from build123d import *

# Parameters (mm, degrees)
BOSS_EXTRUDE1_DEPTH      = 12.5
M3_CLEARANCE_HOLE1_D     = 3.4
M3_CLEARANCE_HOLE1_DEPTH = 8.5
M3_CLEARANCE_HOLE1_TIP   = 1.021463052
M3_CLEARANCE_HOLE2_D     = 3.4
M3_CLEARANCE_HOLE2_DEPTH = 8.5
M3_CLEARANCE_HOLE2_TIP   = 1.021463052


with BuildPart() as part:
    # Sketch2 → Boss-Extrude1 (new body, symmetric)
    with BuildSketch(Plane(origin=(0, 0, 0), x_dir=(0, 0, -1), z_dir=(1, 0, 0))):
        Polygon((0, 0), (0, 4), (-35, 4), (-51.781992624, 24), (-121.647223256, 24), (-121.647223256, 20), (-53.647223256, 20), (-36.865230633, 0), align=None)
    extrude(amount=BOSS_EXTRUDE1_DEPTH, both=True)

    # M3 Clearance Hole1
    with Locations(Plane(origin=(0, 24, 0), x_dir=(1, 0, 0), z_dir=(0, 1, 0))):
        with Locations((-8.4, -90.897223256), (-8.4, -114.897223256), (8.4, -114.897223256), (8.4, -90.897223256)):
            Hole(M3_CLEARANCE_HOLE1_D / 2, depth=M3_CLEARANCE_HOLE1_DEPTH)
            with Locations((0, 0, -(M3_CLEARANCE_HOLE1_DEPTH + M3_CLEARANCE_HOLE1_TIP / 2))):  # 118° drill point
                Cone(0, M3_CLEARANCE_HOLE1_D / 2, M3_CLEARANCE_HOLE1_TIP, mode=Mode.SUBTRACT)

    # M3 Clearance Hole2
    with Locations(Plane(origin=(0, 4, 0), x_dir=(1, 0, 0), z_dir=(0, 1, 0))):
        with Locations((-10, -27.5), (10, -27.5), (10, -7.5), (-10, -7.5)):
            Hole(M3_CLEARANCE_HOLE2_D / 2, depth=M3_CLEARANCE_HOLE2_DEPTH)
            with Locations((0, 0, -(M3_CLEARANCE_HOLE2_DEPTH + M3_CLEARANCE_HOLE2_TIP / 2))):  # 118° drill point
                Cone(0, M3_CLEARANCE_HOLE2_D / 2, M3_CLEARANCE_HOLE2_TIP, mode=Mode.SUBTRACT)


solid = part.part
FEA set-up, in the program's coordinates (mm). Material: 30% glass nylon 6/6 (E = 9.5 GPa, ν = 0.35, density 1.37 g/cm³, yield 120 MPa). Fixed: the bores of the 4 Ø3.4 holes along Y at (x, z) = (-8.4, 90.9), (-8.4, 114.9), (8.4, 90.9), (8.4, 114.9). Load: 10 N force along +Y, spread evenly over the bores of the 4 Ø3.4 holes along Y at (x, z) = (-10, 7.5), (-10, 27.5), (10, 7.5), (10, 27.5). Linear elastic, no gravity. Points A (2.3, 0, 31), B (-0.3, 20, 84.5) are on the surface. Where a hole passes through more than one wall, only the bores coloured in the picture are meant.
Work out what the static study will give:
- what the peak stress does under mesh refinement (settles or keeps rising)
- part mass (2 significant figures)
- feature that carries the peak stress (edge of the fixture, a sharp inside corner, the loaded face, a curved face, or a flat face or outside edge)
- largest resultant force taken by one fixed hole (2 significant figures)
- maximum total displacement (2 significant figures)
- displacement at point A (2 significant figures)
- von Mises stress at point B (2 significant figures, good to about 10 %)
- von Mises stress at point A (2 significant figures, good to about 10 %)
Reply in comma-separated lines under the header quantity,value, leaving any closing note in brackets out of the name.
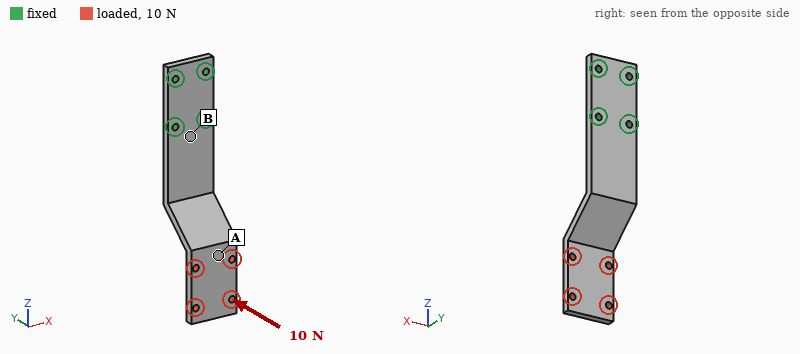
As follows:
quantity,value
what the peak stress does under mesh refinement,keeps rising
part mass,18 g
feature that carries the peak stress,edge of the fixture
largest resultant force taken by one fixed hole,7.6 N
maximum total displacement,1.5 mm
displacement at point A,0.86 mm
von Mises stress at point B,8.7 MPa
von Mises stress at point A,1.9 MPa
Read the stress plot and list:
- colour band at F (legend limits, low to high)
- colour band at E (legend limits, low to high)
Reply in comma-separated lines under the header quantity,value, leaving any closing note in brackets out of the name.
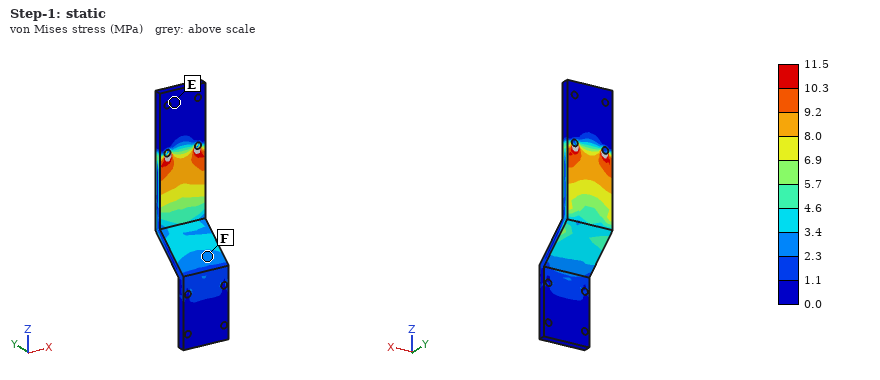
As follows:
quantity,value
colour band at F,2.3 to 3.4 MPa
colour band at E,0.0 to 1.1 MPa
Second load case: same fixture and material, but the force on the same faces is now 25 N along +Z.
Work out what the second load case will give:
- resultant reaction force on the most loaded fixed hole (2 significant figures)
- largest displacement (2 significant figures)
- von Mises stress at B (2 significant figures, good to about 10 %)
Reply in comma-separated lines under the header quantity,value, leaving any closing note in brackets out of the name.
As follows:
quantity,value
resultant reaction force on the most loaded fixed hole,12 N
largest displacement,1.3 mm
von Mises stress at B,6.7 MPa
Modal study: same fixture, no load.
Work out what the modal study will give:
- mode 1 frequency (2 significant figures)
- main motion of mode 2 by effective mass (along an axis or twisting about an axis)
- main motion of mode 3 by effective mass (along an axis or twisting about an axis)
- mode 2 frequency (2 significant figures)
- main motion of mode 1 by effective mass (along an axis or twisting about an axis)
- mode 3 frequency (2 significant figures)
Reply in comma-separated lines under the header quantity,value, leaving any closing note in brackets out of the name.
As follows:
quantity,value
mode 1 frequency,190 Hz
main motion of mode 2 by effective mass,along X
main motion of mode 3 by effective mass,along Y
mode 2 frequency,630 Hz
main motion of mode 1 by effective mass,along Y
mode 3 frequency,1100 Hz
